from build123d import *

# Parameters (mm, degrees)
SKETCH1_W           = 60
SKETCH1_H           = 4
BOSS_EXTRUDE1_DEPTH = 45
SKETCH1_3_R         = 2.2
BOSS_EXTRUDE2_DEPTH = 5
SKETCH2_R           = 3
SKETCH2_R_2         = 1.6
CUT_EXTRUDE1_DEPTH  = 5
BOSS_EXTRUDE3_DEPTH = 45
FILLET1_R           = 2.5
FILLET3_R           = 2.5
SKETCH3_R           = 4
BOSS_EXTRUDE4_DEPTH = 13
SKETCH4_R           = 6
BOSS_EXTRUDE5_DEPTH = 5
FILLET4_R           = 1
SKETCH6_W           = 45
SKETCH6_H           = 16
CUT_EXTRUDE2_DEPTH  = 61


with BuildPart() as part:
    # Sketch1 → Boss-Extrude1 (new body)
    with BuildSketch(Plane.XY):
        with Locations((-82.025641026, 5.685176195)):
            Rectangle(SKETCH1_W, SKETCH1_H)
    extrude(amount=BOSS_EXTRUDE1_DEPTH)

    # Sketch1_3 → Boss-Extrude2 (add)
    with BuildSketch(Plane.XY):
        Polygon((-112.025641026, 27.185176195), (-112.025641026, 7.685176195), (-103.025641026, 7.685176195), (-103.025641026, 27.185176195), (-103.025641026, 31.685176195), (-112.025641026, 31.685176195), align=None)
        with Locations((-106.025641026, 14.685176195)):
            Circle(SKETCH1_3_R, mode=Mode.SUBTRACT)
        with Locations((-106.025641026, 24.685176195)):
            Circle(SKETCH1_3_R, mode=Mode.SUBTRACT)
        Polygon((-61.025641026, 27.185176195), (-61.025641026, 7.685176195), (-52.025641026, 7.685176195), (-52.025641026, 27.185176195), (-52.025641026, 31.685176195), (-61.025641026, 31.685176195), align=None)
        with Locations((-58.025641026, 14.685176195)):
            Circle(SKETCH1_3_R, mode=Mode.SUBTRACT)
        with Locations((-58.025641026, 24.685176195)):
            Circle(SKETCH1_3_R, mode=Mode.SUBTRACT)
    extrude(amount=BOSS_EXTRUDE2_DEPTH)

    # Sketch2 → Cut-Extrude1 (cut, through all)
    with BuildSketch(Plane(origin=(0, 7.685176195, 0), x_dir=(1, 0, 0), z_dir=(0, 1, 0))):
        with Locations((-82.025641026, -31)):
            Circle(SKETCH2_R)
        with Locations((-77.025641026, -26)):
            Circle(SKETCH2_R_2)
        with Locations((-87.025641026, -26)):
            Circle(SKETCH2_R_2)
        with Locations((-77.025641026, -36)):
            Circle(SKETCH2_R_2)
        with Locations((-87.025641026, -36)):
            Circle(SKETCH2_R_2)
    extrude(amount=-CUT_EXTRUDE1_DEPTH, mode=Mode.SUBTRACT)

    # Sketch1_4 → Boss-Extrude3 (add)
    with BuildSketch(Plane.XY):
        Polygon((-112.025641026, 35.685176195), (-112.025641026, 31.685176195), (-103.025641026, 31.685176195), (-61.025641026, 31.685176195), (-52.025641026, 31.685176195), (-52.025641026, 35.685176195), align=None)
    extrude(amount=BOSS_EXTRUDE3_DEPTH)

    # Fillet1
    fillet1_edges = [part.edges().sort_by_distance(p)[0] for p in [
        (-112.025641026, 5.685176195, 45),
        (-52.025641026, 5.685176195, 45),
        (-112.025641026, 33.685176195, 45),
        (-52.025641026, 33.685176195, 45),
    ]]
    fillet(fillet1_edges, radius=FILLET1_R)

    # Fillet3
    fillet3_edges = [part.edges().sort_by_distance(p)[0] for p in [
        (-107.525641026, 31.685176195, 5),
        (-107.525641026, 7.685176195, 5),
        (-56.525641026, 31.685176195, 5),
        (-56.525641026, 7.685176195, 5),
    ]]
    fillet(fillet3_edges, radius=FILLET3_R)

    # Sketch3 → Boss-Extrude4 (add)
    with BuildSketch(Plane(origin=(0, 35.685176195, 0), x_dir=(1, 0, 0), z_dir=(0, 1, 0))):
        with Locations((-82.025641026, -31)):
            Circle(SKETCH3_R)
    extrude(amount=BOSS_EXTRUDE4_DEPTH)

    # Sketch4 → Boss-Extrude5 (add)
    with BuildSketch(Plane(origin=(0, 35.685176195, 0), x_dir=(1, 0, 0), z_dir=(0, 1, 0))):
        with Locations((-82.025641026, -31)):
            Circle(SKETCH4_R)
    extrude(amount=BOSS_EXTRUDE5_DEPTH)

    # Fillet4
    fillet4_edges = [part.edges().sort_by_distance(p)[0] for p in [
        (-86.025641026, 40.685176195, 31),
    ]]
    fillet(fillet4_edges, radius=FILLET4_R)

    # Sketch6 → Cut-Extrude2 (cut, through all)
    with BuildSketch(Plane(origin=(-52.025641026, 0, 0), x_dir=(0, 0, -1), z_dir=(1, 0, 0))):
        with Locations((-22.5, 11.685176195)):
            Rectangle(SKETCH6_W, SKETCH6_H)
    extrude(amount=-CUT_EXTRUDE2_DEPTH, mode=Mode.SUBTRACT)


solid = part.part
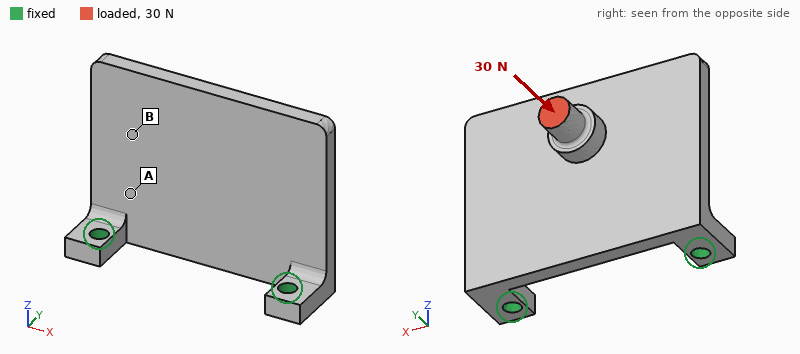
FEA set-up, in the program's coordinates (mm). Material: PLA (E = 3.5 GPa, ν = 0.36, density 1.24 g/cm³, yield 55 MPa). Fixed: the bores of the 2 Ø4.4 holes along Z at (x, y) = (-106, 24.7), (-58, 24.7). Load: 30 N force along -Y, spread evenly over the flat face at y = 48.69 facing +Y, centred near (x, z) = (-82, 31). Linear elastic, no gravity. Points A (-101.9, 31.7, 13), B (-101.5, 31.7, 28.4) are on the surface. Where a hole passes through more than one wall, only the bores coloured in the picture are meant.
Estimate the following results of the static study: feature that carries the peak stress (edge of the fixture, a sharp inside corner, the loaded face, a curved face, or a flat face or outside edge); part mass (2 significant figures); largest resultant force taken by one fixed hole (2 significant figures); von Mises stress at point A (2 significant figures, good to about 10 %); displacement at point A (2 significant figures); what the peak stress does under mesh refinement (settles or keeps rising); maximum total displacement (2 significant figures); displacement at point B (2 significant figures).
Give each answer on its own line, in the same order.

a sharp inside corner
16 g
17 N
4.2 MPa
0.14 mm
keeps rising
0.89 mm
0.46 mm
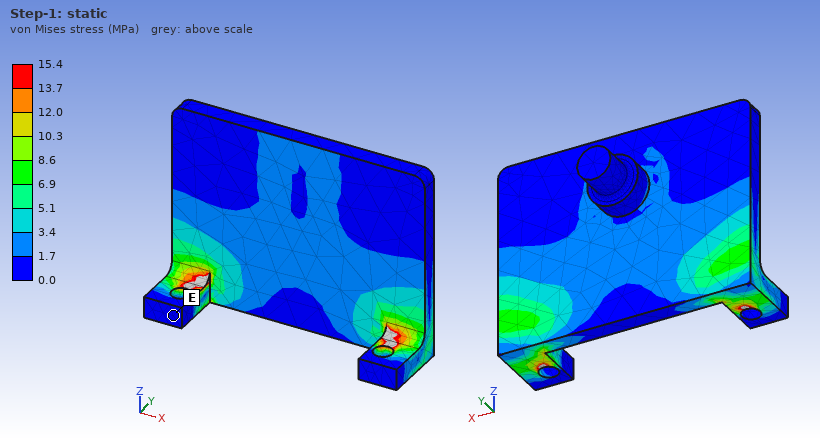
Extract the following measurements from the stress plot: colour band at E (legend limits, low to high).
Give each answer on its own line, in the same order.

0.0 to 1.7 MPa
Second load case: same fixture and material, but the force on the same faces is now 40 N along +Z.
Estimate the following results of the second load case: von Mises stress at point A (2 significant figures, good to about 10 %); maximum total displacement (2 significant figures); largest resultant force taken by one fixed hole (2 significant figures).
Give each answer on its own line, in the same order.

4.0 MPa
0.87 mm
21 N
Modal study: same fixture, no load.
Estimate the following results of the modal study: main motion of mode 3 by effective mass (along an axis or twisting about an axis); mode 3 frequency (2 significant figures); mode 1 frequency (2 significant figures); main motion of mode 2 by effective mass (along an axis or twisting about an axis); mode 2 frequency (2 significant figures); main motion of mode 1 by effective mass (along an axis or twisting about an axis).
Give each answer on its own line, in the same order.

along X
2000 Hz
360 Hz
twisting about Z
1100 Hz
along Y
